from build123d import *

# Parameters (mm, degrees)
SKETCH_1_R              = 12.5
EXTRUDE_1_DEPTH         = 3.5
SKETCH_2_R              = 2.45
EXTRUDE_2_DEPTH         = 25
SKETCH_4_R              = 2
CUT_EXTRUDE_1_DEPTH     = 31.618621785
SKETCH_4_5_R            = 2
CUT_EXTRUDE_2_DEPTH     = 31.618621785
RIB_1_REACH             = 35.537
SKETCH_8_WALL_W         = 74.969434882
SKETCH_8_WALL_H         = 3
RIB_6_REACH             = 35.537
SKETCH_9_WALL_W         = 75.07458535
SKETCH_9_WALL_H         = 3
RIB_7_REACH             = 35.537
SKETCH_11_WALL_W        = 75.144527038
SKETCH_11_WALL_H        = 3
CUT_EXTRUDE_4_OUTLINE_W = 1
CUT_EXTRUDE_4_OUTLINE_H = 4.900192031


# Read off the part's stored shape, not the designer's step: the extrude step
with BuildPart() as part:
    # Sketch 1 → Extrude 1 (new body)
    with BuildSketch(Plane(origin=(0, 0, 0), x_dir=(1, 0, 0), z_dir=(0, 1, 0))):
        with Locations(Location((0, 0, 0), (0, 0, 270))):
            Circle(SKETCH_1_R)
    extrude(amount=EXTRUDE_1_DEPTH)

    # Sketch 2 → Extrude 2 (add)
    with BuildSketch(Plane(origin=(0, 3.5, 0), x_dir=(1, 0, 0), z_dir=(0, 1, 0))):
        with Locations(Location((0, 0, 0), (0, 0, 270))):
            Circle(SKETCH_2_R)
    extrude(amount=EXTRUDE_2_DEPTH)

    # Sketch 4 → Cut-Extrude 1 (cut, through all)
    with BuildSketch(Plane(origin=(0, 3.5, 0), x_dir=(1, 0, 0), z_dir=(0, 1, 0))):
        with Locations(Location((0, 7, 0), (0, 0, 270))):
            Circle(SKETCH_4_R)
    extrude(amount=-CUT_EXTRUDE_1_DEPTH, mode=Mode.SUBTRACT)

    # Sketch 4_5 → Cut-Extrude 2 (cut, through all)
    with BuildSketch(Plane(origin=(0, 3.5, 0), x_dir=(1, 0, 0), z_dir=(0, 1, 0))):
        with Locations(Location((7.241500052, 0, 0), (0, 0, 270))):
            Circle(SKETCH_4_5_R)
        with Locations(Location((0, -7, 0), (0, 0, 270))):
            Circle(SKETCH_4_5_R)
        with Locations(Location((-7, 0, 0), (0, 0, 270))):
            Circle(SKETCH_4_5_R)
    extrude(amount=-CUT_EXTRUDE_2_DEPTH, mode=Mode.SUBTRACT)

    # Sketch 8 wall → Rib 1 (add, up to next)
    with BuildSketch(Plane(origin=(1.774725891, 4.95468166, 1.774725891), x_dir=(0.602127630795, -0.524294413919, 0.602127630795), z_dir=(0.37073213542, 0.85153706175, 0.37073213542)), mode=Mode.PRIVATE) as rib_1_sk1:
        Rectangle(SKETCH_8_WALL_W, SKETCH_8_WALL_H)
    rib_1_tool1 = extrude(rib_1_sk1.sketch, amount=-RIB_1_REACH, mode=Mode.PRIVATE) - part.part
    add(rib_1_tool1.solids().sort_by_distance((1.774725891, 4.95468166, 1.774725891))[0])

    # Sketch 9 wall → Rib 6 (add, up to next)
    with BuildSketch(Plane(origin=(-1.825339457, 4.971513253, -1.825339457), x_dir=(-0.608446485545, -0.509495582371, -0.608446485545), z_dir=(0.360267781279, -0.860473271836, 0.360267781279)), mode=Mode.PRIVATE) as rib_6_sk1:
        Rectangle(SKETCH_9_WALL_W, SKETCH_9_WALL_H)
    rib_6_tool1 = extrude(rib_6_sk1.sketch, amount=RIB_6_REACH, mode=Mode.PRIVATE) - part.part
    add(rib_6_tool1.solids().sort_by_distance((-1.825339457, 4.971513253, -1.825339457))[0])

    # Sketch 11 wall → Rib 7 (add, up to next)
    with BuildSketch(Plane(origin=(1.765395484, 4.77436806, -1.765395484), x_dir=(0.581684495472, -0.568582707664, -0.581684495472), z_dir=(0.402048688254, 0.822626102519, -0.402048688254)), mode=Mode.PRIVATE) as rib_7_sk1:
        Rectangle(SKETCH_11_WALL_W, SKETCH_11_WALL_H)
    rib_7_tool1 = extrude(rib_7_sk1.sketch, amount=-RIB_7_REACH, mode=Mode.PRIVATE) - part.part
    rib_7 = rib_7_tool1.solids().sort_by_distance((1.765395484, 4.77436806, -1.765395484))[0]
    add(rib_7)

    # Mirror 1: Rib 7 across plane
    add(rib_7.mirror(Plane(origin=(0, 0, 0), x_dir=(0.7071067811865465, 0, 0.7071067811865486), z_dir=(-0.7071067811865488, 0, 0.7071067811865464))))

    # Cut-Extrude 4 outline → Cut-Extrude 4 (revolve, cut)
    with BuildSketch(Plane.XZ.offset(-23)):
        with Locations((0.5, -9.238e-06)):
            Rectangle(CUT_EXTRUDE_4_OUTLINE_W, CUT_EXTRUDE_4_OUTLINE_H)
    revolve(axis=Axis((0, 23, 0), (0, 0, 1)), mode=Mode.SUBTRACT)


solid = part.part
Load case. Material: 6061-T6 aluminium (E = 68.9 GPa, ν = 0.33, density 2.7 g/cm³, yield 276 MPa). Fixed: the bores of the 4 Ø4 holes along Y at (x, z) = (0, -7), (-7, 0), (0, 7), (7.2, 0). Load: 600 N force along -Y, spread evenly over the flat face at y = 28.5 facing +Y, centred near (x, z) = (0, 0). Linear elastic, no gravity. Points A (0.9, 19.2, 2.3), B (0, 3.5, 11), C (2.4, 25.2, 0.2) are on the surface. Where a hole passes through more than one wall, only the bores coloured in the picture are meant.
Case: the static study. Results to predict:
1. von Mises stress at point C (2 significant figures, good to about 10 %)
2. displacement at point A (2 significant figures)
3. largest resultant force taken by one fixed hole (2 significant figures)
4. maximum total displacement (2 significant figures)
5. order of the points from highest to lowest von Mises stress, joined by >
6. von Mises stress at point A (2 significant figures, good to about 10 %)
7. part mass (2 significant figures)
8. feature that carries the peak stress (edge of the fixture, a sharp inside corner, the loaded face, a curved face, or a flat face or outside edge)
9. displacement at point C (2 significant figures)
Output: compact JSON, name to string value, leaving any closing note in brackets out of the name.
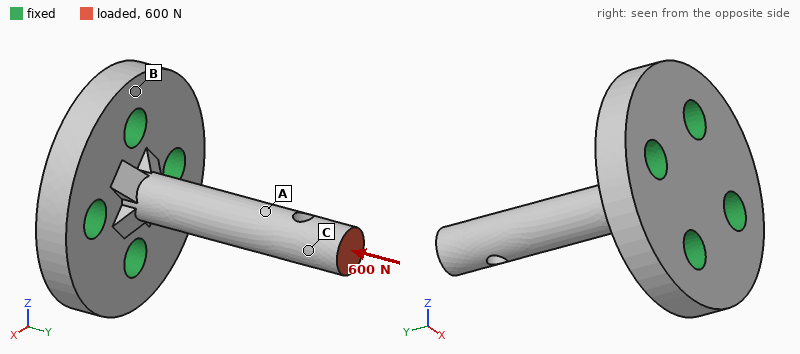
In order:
{"von Mises stress at point C": "50 MPa", "displacement at point A": "8.4 µm", "largest resultant force taken by one fixed hole": "170 N", "maximum total displacement": "14 µm", "order of the points from highest to lowest von Mises stress, joined by >": "C > A > B", "von Mises stress at point A": "29 MPa", "part mass": "5.5 g", "feature that carries the peak stress": "a curved face", "displacement at point C": "12 µm"}
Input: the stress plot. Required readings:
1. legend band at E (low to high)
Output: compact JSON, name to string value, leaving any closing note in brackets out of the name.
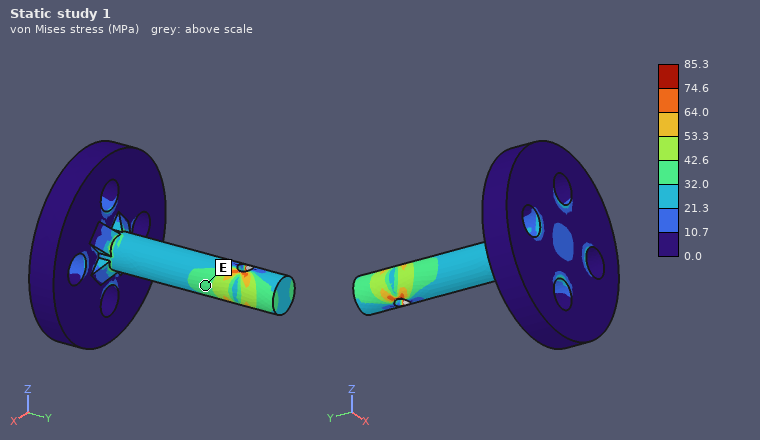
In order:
{"legend band at E": "32.0 to 42.6 MPa"}
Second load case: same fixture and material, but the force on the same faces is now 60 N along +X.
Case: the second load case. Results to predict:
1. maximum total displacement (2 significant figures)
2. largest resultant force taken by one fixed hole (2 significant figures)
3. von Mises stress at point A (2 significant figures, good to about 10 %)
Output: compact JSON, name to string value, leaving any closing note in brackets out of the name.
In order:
{"maximum total displacement": "0.17 mm", "largest resultant force taken by one fixed hole": "140 N", "von Mises stress at point A": "19 MPa"}
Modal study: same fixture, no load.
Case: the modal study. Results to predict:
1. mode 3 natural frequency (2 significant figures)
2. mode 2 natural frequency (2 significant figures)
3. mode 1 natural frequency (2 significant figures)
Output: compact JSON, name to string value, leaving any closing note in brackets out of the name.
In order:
{"mode 3 natural frequency": "29 kHz", "mode 2 natural frequency": "5600 Hz", "mode 1 natural frequency": "5600 Hz"}
